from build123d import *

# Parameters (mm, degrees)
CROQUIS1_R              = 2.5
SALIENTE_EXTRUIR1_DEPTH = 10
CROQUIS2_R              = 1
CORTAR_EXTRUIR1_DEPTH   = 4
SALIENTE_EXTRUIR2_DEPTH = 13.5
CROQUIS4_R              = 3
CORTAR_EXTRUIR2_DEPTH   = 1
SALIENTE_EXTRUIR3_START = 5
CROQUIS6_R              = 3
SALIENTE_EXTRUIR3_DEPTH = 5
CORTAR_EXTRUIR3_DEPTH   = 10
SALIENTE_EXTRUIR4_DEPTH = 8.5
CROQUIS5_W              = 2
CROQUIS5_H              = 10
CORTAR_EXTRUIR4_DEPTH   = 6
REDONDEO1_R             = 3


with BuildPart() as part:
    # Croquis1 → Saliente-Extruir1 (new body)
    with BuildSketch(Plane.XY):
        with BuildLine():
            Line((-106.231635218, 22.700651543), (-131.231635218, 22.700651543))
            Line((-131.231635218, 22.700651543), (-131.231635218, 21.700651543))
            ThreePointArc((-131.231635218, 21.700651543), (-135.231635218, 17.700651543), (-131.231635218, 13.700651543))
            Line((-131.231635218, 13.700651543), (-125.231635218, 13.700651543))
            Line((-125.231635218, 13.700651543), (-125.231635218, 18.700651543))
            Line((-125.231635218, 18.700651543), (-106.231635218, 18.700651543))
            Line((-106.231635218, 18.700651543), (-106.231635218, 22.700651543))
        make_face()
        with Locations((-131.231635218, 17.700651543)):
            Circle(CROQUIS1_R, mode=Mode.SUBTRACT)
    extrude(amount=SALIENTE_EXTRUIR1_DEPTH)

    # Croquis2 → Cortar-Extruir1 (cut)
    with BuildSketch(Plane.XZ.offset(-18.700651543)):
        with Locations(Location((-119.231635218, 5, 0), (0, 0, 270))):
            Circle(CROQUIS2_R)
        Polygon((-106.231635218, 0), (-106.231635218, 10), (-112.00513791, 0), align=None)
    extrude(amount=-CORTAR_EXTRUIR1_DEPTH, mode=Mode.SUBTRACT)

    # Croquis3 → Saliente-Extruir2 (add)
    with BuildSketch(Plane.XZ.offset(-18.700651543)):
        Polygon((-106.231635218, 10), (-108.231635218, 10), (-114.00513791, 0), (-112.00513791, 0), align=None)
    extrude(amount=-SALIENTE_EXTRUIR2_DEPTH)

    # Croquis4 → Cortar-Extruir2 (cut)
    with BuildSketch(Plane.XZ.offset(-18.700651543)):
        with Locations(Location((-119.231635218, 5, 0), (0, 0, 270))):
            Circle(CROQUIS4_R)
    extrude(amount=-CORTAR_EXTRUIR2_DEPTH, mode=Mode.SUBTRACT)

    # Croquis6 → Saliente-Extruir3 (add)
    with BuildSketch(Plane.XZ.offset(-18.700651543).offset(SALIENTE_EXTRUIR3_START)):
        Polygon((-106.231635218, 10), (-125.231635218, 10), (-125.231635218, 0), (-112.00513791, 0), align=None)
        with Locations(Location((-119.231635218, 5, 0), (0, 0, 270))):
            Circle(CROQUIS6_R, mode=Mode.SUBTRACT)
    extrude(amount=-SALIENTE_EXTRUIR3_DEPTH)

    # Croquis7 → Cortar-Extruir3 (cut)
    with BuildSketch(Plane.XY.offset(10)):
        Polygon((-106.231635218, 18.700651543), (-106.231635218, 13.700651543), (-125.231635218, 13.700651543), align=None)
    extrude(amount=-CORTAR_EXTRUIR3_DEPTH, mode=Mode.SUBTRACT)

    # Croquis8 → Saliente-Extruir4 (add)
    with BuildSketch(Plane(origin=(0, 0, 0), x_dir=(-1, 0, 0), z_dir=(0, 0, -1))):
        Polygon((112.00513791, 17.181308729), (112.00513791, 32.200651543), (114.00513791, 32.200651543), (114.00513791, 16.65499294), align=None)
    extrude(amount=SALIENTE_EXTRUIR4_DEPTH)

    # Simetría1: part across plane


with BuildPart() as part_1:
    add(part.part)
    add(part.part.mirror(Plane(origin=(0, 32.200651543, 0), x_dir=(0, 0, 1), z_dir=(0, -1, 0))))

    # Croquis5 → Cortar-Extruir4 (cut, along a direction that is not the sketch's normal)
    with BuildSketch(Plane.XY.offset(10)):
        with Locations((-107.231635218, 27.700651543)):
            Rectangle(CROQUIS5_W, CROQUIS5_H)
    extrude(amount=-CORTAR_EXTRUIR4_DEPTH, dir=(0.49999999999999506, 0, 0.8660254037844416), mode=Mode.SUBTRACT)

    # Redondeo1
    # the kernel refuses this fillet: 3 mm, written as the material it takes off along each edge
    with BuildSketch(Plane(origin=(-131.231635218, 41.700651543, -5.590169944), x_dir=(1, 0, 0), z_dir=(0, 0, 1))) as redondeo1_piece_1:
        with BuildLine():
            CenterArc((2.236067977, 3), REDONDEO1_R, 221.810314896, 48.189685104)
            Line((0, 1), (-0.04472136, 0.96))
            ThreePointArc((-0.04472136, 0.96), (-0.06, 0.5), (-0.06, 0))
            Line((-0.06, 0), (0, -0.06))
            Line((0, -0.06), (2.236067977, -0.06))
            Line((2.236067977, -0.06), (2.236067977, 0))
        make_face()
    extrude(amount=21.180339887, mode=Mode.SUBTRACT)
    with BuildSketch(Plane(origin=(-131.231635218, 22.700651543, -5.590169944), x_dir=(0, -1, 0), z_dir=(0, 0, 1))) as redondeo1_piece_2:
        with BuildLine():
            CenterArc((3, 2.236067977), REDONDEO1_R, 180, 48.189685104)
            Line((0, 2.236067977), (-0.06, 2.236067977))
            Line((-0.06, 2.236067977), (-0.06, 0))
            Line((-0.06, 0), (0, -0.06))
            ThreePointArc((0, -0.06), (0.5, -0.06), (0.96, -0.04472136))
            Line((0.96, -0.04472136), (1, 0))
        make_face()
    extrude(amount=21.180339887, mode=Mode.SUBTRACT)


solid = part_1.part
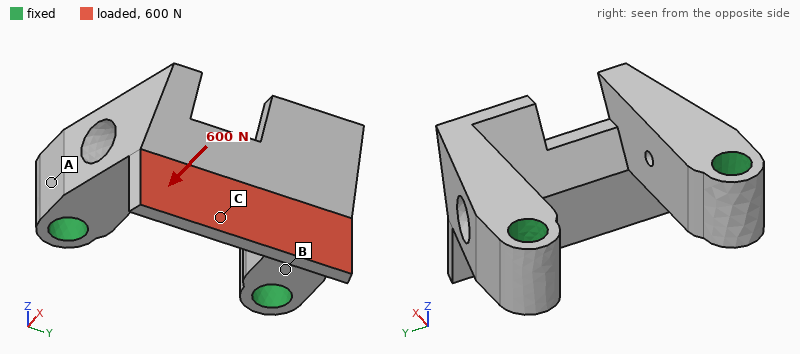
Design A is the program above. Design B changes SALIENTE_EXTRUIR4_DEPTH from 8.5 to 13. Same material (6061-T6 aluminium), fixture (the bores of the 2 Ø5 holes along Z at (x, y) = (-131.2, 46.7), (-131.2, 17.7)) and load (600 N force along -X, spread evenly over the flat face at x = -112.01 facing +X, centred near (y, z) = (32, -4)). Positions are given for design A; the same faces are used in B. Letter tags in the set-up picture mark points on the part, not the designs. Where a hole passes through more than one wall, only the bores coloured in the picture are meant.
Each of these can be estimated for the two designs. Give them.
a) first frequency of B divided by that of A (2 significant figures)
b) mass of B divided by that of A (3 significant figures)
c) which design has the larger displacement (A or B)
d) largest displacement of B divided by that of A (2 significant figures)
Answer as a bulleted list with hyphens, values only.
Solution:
- 0.59
- 1.07
- B
- 2.1
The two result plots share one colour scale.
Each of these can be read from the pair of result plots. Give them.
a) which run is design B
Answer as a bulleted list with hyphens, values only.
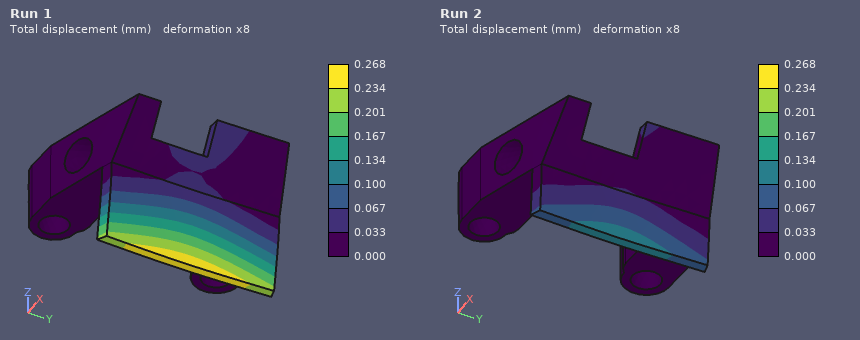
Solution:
- Run 1
